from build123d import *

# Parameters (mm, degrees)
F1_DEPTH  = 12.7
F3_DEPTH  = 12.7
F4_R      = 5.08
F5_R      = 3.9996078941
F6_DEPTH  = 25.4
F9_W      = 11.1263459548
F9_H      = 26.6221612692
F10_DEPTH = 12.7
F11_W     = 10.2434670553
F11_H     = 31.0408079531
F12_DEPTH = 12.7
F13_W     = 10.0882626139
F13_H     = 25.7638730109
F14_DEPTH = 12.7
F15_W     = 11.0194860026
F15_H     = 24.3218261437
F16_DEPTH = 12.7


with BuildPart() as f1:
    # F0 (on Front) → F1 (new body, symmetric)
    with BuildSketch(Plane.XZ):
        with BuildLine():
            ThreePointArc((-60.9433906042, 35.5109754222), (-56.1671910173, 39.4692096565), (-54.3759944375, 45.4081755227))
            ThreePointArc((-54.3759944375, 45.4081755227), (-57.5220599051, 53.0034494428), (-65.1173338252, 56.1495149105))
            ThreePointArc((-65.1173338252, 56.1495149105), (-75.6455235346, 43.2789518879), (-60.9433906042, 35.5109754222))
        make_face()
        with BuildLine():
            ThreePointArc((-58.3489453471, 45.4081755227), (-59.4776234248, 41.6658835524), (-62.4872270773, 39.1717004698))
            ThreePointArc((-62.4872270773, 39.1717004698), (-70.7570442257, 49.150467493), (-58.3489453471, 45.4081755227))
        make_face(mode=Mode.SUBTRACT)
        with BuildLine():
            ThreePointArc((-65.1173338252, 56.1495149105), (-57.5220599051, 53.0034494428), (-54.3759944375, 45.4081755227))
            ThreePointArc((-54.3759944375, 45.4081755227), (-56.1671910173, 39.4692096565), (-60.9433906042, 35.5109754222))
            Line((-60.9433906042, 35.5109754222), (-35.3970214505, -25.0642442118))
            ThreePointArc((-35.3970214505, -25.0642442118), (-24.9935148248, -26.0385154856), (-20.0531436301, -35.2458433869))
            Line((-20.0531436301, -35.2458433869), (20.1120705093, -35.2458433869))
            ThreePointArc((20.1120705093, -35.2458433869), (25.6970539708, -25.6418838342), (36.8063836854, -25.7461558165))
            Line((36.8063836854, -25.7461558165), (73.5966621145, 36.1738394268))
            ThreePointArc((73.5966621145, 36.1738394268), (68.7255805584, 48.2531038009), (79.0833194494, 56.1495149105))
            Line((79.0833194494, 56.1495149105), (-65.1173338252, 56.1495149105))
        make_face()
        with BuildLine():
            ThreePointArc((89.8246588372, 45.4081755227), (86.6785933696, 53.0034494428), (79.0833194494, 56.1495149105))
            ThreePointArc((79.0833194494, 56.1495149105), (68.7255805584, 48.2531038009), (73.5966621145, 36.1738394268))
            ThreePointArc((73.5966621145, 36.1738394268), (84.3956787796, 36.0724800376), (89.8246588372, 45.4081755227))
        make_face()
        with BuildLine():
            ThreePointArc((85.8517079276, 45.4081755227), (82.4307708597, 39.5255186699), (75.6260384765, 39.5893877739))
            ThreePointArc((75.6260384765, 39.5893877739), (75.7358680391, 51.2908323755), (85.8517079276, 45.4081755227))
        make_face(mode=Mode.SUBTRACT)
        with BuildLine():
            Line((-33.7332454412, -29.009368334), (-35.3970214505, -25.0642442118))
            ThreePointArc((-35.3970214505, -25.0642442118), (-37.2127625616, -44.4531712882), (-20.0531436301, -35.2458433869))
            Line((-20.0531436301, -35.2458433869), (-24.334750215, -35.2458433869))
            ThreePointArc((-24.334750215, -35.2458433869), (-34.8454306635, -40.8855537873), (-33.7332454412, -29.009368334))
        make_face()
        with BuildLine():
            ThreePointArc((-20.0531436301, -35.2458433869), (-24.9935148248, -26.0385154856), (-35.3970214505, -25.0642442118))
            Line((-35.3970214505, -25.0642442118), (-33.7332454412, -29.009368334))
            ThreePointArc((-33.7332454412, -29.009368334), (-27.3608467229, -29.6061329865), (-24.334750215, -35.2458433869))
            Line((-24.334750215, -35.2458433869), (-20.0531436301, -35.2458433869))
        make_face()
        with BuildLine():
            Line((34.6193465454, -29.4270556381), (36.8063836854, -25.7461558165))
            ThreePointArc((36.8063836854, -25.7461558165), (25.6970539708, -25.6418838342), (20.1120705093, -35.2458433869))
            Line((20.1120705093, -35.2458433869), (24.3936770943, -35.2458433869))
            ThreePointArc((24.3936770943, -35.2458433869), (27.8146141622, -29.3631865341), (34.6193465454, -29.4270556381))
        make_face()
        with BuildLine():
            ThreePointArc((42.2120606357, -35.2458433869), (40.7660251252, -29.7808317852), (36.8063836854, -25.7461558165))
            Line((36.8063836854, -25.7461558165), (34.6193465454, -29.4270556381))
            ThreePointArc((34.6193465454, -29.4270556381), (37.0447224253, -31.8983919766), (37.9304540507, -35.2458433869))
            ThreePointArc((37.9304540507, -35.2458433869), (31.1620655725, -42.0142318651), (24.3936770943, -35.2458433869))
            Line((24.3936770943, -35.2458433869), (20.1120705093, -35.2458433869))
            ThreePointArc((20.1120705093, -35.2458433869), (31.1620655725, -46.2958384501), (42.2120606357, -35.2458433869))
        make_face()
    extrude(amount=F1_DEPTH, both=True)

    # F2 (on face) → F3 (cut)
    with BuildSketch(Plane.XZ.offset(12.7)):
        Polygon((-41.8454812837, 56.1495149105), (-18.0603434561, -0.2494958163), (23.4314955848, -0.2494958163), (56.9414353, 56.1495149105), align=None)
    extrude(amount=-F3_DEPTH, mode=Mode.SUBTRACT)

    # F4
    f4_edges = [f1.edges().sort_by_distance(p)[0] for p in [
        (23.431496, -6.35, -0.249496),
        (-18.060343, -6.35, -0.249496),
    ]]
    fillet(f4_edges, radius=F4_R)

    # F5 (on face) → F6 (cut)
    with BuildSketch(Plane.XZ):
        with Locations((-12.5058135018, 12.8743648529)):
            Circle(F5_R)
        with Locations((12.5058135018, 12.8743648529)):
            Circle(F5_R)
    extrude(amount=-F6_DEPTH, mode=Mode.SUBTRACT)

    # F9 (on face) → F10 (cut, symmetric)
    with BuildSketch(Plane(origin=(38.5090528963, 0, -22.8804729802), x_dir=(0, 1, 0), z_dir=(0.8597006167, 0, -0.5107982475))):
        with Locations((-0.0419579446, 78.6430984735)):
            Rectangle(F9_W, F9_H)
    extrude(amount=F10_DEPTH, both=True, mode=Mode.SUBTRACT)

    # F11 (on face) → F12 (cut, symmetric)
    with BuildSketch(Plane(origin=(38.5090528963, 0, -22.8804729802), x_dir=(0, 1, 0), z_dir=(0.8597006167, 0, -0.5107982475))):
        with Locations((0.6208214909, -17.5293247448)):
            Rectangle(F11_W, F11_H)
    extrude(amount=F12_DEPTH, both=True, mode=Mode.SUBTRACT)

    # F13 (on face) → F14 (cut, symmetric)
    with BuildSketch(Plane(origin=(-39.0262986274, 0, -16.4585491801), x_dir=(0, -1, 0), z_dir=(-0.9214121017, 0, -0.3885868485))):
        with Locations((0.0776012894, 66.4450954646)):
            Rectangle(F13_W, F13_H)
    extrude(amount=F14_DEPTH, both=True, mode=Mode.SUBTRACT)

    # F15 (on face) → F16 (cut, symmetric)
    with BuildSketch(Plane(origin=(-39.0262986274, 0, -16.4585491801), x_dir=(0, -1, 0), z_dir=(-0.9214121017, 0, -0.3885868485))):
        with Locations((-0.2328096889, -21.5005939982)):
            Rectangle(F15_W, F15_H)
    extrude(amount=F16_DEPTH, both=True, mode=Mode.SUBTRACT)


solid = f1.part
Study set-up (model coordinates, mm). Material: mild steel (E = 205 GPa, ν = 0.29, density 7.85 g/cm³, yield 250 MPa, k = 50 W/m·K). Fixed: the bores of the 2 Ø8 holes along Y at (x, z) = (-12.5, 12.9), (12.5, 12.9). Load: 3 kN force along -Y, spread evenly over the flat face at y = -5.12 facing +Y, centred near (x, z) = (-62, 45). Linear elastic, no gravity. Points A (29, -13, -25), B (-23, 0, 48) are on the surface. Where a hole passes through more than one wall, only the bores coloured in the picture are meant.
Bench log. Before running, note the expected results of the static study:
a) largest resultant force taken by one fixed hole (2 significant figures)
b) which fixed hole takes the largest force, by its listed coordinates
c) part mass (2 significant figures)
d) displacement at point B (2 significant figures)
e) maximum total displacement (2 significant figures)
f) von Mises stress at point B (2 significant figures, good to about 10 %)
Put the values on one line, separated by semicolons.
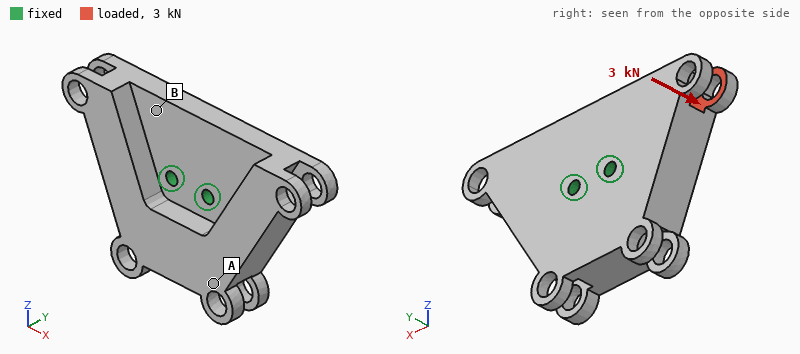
5.9 kN; (-12.5, 12.9); 1.5 kg; 0.020 mm; 0.12 mm; 25 MPa
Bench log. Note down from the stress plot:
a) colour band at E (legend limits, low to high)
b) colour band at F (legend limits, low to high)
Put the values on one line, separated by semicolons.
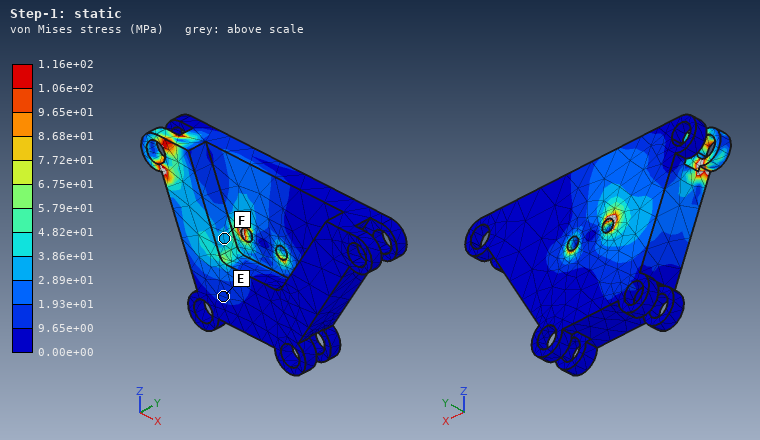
9.65e+00 to 1.93e+01 MPa; 2.89e+01 to 3.86e+01 MPa
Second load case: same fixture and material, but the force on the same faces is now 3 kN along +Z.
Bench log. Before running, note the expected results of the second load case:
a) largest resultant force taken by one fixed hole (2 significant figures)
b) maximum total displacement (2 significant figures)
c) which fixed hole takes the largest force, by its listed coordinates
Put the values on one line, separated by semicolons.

7.4 kN; 39 µm; (-12.5, 12.9)
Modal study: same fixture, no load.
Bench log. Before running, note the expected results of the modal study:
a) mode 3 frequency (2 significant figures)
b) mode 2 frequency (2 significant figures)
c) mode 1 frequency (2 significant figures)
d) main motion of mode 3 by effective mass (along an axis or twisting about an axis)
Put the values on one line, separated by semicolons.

3800 Hz; 2900 Hz; 2400 Hz; twisting about Y
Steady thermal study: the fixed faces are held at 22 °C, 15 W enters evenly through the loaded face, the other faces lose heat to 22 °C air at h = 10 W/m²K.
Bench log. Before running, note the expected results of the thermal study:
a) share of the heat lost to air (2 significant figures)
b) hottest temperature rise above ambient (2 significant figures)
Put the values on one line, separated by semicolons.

13 %; 54 K
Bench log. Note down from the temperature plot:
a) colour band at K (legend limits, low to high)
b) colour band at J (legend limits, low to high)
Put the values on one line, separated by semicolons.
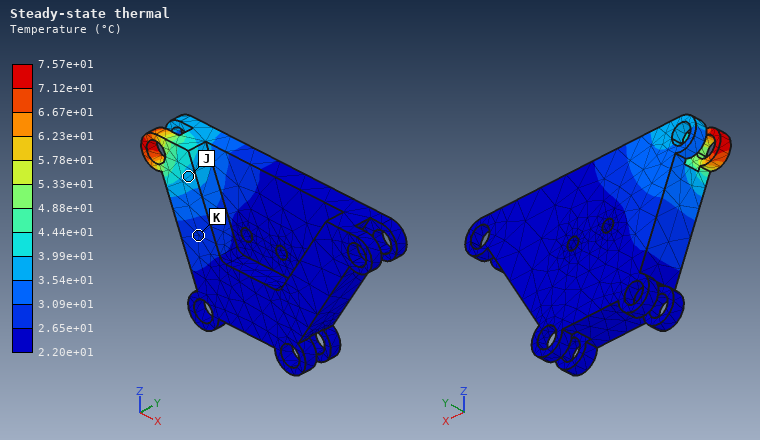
2.65e+01 to 3.09e+01 °C; 3.54e+01 to 3.99e+01 °C
